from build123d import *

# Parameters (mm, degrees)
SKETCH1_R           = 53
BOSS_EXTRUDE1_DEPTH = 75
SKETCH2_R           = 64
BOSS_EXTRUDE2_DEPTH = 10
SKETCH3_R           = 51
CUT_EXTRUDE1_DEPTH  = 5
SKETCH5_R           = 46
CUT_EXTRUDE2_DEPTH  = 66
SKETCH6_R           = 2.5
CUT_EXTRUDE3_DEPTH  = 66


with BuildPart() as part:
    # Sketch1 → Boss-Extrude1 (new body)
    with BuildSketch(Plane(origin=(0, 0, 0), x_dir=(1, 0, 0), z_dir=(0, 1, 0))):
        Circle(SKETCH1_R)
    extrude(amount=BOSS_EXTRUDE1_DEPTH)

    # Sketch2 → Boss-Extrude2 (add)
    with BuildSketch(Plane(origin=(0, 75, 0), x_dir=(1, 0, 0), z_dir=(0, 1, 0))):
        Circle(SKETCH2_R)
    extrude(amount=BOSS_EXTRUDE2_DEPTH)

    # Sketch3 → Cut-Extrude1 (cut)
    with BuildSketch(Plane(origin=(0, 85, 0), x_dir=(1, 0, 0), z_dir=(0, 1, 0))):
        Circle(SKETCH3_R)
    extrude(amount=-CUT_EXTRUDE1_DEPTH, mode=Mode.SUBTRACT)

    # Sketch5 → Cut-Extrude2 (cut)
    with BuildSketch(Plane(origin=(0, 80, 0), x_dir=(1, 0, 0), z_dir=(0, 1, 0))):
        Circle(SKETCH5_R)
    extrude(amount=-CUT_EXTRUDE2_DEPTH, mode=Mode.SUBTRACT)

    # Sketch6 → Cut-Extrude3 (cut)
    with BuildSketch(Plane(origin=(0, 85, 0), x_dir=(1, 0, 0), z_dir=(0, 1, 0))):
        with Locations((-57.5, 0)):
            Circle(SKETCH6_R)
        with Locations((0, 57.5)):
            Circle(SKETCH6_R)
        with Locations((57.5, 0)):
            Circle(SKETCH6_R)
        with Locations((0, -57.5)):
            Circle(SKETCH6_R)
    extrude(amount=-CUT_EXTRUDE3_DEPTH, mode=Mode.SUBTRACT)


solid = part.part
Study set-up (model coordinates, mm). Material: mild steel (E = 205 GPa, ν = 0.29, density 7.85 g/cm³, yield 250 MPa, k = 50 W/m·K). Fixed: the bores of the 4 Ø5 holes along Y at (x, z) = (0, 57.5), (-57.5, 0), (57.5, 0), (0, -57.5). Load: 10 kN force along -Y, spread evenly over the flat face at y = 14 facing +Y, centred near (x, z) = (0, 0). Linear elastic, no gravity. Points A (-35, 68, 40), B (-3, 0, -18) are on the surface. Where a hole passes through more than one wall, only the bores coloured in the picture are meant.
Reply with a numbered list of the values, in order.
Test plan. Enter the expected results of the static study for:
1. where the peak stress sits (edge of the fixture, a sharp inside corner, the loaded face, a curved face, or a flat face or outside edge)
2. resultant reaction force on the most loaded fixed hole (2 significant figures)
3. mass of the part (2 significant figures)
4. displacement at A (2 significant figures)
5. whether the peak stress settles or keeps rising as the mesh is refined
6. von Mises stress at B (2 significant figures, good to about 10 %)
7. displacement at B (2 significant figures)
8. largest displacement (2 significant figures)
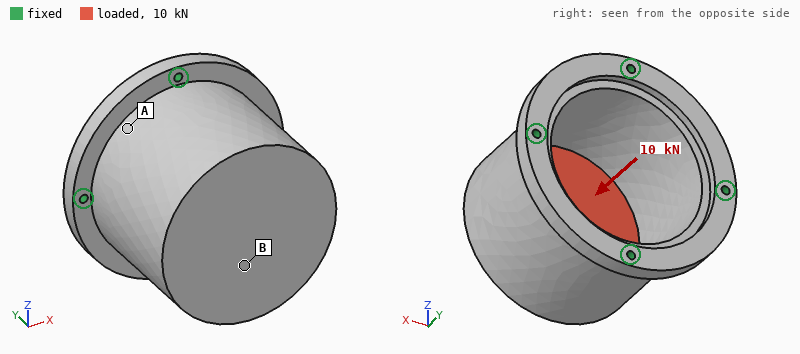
1. edge of the fixture
2. 2.6 kN
3. 2.4 kg
4. 3.7 µm
5. keeps rising
6. 14 MPa
7. 11 µm
8. 12 µm
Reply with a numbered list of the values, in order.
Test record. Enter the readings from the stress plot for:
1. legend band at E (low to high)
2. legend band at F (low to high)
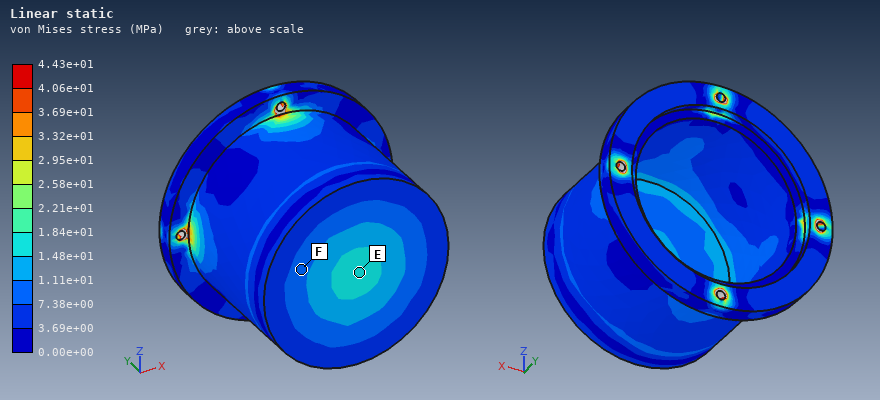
1. 1.48e+01 to 1.84e+01 MPa
2. 7.38e+00 to 1.11e+01 MPa
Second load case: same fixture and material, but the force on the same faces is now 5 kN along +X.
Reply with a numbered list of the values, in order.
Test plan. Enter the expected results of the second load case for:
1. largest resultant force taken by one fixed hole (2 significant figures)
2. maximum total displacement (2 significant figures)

1. 3.1 kN
2. 12 µm
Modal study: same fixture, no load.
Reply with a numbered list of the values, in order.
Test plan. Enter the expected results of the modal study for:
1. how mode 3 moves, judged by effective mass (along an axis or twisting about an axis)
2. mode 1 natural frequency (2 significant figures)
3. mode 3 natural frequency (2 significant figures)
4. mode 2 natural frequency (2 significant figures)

1. along Y
2. 2900 Hz
3. 5000 Hz
4. 2900 Hz
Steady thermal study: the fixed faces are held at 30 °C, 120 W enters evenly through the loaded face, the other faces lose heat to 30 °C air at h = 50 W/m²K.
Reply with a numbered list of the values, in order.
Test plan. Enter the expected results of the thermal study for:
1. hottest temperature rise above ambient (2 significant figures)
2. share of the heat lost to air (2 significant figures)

1. 59 K
2. 70 %
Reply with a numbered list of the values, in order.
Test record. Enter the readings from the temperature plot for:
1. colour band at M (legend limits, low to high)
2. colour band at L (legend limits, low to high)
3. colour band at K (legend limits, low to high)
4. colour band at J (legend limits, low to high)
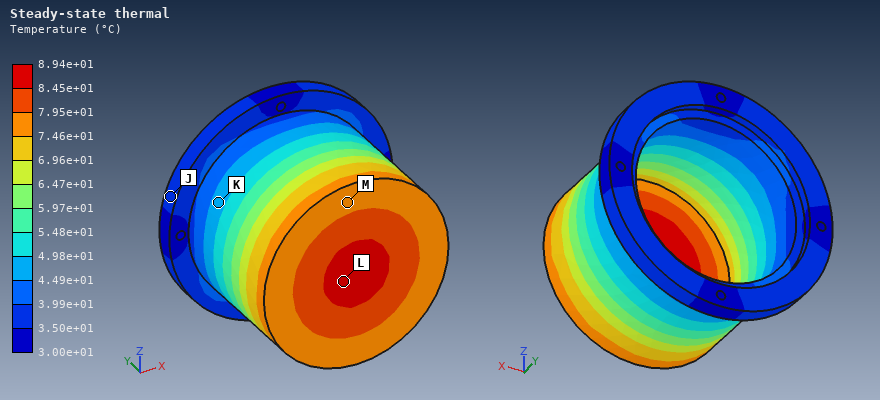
1. 7.46e+01 to 7.95e+01 °C
2. 8.45e+01 to 8.94e+01 °C
3. 4.49e+01 to 4.98e+01 °C
4. 3.50e+01 to 3.99e+01 °C
